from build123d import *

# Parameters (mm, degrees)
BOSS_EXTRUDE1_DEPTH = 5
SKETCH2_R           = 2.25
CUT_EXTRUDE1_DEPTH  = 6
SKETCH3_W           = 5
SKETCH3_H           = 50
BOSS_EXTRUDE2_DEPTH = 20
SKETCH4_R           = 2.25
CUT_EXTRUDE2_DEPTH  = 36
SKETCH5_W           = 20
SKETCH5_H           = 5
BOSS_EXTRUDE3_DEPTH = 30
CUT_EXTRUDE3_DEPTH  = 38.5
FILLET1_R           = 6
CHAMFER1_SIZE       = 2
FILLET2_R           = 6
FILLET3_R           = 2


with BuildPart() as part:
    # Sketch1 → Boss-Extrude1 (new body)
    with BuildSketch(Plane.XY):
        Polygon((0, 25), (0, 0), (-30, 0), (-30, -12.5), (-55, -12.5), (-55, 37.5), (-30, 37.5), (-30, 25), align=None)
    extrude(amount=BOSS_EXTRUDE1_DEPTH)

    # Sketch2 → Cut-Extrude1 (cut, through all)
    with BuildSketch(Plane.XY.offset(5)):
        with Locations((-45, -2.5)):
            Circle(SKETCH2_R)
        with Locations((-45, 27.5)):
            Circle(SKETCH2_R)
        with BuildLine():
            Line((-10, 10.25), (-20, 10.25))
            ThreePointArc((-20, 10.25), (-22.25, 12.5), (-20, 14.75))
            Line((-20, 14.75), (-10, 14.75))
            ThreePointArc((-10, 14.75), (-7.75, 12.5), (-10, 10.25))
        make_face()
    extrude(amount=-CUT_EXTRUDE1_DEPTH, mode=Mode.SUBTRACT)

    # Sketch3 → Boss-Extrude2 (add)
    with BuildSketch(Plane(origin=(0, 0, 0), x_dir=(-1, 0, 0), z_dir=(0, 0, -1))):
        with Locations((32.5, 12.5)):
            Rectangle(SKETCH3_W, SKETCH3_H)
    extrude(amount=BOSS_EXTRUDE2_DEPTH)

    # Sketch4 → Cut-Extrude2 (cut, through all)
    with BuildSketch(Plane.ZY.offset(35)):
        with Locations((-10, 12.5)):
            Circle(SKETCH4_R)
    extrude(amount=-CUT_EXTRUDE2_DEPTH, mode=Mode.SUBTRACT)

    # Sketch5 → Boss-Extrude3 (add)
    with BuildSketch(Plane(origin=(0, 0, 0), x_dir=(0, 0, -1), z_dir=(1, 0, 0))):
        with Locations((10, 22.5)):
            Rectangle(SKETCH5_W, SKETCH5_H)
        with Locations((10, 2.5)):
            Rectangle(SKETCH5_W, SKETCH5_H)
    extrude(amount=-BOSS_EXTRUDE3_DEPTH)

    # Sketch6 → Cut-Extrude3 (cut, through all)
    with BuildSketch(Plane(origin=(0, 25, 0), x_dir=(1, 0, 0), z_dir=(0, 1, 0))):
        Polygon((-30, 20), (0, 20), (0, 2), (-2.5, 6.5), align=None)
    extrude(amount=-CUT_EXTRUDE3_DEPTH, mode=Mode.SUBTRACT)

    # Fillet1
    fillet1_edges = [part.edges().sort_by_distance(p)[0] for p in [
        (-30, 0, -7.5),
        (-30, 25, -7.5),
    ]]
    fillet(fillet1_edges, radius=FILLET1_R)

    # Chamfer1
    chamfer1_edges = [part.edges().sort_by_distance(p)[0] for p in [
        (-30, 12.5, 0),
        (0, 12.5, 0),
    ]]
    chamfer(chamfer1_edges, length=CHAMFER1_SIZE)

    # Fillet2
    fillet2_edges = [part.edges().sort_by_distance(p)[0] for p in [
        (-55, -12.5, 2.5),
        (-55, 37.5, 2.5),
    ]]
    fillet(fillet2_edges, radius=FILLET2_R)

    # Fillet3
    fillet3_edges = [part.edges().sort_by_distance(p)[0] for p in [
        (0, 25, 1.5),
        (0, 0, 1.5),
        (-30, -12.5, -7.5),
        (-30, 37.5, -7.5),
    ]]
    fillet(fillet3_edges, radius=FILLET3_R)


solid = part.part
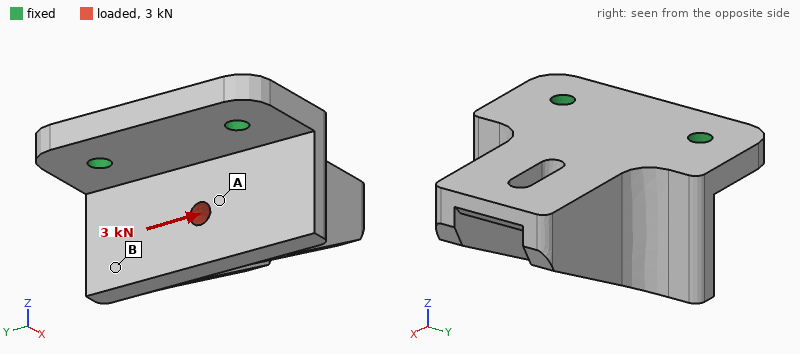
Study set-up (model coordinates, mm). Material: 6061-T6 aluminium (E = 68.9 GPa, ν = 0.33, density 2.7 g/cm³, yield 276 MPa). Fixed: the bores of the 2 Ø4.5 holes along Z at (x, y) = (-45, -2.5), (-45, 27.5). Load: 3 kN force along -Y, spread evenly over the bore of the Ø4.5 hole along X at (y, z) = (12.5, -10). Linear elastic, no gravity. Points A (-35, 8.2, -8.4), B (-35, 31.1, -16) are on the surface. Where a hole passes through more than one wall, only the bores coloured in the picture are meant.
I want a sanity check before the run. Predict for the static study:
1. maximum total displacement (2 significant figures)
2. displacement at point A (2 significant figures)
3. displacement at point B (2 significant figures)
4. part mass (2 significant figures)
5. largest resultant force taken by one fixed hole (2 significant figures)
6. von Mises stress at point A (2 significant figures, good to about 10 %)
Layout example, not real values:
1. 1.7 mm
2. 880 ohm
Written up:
1. 68 µm
2. 33 µm
3. 54 µm
4. 50 g
5. 2.2 kN
6. 49 MPa
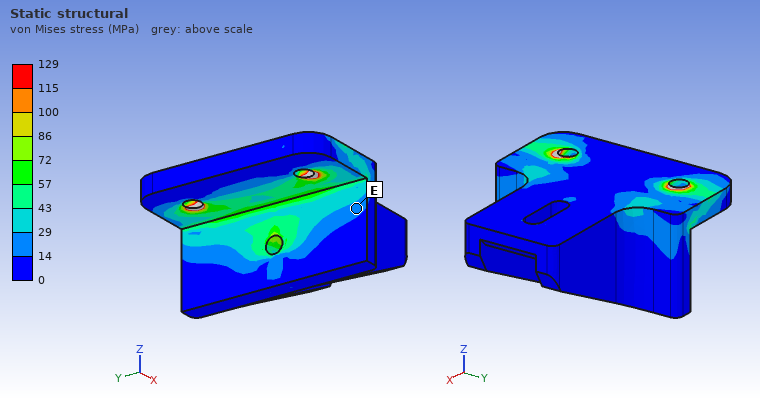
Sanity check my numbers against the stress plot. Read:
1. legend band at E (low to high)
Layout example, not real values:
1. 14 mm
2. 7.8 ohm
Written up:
1. 14 to 29 MPa
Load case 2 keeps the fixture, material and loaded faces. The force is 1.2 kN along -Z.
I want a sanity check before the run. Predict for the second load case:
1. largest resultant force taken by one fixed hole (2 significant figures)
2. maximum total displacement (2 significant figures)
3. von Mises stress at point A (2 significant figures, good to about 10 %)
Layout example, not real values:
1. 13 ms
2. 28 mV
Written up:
1. 600 N
2. 0.12 mm
3. 11 MPa
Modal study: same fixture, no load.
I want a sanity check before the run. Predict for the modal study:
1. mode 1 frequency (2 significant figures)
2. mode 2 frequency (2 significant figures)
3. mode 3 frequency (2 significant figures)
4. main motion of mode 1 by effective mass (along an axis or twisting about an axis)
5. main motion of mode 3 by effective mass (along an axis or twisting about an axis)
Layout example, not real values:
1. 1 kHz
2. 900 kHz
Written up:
1. 2000 Hz
2. 6800 Hz
3. 9100 Hz
4. along Z
5. along Y
